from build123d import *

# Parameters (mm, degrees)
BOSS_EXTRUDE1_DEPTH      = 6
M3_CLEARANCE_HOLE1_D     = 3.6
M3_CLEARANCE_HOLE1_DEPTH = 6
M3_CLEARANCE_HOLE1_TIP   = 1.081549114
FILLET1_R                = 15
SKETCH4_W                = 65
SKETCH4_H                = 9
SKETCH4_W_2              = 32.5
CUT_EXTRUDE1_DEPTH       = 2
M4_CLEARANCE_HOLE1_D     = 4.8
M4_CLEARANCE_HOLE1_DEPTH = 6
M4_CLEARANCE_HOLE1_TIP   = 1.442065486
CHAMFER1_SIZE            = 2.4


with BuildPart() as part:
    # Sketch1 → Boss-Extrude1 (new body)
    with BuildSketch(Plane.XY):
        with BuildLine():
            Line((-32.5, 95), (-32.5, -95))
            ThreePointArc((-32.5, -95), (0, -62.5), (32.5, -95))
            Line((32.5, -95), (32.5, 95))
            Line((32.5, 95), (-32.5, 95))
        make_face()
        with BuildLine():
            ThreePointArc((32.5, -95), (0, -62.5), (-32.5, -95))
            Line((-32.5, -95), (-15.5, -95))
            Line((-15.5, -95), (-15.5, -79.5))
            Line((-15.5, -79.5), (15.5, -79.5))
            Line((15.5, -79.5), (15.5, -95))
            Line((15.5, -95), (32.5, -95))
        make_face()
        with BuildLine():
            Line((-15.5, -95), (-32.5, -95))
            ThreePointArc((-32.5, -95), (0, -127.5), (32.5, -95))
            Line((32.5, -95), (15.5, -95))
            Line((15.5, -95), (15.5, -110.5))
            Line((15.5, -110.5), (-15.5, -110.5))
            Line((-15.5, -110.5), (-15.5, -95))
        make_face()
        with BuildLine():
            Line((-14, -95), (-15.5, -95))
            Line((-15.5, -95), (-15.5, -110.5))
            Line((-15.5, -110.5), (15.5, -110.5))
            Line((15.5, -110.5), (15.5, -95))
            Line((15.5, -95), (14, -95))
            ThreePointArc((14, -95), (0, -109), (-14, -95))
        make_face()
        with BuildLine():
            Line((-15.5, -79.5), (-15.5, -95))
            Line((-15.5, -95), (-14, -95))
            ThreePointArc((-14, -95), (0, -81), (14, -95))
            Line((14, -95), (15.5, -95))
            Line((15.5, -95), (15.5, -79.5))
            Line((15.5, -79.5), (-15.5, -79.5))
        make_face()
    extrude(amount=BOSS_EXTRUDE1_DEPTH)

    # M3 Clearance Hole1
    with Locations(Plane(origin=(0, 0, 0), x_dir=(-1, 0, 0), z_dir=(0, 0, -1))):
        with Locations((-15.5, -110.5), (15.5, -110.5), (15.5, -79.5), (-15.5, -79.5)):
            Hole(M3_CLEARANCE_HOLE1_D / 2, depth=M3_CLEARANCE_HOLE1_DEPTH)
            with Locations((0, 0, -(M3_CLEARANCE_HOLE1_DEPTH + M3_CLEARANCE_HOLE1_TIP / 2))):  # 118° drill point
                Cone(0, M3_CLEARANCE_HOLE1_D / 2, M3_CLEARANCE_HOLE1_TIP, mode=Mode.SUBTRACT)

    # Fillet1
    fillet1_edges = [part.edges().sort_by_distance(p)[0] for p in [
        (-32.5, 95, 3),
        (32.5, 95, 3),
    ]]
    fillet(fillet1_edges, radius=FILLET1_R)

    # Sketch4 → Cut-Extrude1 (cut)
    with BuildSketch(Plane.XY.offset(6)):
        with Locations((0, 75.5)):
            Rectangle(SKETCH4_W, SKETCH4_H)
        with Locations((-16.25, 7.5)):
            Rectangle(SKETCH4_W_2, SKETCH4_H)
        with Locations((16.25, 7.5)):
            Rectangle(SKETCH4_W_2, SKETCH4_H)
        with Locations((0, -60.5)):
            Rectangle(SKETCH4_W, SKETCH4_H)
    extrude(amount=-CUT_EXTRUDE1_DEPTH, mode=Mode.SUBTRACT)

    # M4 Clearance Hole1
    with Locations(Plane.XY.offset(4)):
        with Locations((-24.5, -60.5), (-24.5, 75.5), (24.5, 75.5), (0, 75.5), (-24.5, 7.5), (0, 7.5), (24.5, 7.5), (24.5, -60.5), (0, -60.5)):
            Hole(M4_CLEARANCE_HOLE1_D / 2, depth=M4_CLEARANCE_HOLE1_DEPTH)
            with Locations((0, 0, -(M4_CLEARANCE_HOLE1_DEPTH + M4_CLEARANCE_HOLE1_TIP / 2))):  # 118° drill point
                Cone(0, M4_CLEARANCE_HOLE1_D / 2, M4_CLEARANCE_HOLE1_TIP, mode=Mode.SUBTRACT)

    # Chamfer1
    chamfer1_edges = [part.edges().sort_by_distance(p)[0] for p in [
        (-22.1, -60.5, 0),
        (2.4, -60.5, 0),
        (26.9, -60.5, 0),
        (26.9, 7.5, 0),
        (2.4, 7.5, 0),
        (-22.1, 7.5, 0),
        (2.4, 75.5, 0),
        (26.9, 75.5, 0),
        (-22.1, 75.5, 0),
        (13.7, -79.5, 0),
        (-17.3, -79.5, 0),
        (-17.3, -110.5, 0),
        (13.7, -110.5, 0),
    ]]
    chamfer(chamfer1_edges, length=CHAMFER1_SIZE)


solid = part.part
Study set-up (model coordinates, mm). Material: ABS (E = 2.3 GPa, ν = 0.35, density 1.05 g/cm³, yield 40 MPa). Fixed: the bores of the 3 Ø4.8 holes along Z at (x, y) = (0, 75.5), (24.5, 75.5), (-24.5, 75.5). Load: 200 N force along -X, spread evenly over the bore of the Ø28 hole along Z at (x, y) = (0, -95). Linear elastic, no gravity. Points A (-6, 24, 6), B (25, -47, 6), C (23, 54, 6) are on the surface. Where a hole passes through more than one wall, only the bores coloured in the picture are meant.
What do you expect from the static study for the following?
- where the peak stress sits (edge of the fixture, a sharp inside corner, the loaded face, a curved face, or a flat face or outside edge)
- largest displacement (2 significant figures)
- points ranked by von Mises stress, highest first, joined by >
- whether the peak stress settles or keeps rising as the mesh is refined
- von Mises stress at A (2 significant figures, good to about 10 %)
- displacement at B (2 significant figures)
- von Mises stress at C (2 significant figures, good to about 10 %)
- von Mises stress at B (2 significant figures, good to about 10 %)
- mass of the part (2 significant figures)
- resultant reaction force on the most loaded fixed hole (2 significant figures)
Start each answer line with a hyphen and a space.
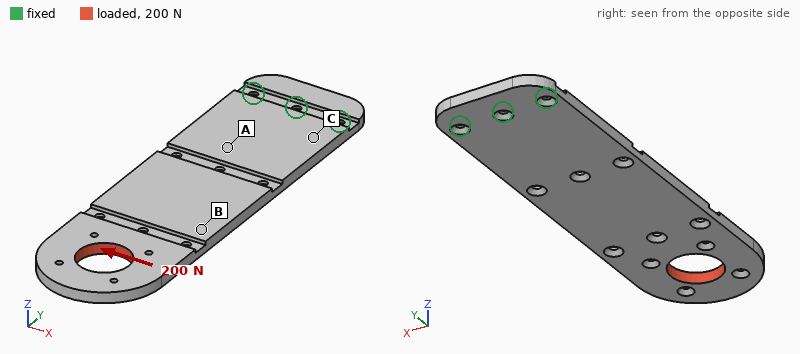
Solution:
- edge of the fixture
- 2.0 mm
- C > A > B
- keeps rising
- 2.4 MPa
- 0.98 mm
- 4.6 MPa
- 1.3 MPa
- 78 g
- 680 N
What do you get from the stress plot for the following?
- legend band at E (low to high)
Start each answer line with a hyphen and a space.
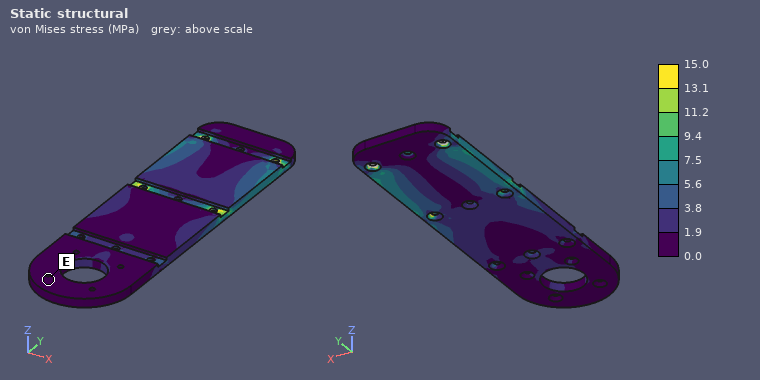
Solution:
- 0.0 to 1.9 MPa
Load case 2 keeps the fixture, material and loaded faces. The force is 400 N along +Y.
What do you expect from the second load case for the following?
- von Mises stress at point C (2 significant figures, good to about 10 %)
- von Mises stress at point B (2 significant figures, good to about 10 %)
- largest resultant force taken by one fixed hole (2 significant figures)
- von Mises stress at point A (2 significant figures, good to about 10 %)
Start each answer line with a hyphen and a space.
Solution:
- 1.0 MPa
- 0.94 MPa
- 140 N
- 1.1 MPa
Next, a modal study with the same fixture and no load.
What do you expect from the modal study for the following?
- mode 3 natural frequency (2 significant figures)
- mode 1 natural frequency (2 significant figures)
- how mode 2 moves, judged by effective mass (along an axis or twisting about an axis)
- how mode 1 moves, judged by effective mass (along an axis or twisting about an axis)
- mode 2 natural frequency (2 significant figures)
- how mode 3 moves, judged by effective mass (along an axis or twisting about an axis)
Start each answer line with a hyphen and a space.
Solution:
- 210 Hz
- 30 Hz
- along Z
- along Z
- 170 Hz
- twisting about Y
